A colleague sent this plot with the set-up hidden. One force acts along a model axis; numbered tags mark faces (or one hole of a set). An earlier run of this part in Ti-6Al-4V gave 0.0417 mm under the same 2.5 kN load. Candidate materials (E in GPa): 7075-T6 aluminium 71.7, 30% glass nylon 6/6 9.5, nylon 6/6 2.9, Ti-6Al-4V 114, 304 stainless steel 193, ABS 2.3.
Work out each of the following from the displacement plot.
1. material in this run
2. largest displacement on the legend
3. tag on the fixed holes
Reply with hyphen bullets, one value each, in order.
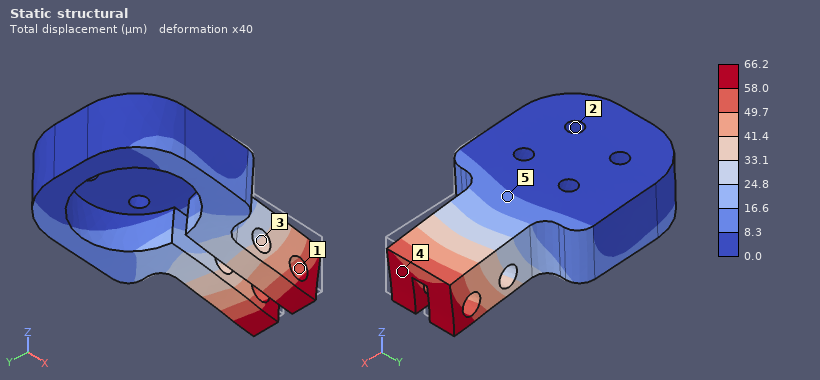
- 7075-T6 aluminium
- 66.2 µm
- 2
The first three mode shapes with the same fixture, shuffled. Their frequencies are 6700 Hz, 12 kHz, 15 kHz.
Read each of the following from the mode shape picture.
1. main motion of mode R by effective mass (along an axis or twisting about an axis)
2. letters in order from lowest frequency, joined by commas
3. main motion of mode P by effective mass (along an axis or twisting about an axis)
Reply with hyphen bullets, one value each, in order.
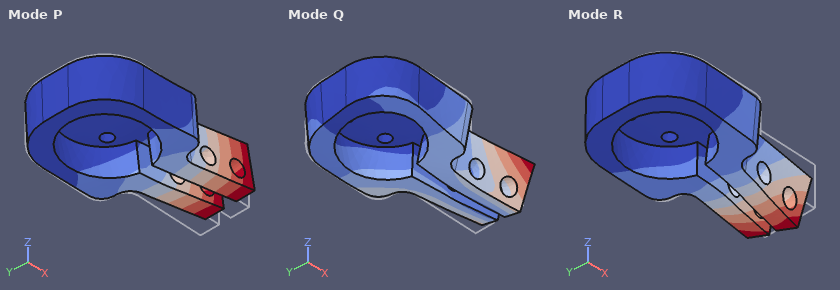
- along Y
- P, R, Q
- along Z
